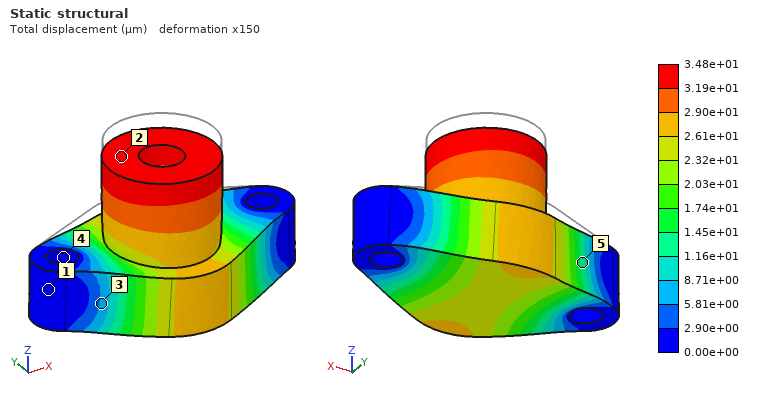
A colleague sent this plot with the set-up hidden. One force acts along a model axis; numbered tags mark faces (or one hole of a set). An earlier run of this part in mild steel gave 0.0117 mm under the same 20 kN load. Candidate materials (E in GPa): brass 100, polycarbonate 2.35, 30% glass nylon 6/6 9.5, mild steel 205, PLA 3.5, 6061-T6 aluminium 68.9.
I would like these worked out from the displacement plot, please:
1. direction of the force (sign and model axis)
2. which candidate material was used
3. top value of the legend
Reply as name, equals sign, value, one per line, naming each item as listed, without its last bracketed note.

direction of the force = -Z
which candidate material was used = 6061-T6 aluminium
top value of the legend = 3.48e+01 µm
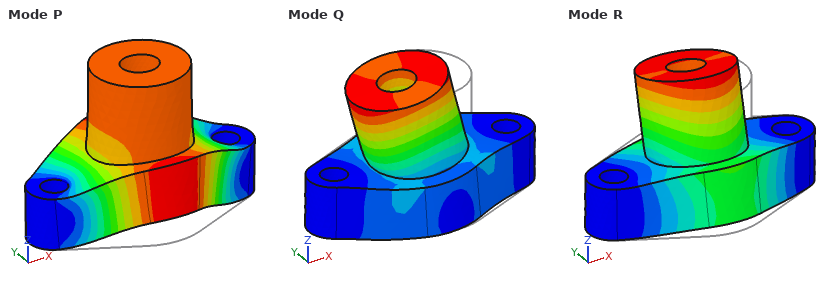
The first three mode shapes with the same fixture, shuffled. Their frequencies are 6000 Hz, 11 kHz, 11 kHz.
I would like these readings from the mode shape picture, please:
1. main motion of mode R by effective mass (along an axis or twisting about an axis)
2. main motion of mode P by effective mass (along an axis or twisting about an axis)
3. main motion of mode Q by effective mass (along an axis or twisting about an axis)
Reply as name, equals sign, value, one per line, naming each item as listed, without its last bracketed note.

main motion of mode R by effective mass = along Y
main motion of mode P by effective mass = along Z
main motion of mode Q by effective mass = along X
